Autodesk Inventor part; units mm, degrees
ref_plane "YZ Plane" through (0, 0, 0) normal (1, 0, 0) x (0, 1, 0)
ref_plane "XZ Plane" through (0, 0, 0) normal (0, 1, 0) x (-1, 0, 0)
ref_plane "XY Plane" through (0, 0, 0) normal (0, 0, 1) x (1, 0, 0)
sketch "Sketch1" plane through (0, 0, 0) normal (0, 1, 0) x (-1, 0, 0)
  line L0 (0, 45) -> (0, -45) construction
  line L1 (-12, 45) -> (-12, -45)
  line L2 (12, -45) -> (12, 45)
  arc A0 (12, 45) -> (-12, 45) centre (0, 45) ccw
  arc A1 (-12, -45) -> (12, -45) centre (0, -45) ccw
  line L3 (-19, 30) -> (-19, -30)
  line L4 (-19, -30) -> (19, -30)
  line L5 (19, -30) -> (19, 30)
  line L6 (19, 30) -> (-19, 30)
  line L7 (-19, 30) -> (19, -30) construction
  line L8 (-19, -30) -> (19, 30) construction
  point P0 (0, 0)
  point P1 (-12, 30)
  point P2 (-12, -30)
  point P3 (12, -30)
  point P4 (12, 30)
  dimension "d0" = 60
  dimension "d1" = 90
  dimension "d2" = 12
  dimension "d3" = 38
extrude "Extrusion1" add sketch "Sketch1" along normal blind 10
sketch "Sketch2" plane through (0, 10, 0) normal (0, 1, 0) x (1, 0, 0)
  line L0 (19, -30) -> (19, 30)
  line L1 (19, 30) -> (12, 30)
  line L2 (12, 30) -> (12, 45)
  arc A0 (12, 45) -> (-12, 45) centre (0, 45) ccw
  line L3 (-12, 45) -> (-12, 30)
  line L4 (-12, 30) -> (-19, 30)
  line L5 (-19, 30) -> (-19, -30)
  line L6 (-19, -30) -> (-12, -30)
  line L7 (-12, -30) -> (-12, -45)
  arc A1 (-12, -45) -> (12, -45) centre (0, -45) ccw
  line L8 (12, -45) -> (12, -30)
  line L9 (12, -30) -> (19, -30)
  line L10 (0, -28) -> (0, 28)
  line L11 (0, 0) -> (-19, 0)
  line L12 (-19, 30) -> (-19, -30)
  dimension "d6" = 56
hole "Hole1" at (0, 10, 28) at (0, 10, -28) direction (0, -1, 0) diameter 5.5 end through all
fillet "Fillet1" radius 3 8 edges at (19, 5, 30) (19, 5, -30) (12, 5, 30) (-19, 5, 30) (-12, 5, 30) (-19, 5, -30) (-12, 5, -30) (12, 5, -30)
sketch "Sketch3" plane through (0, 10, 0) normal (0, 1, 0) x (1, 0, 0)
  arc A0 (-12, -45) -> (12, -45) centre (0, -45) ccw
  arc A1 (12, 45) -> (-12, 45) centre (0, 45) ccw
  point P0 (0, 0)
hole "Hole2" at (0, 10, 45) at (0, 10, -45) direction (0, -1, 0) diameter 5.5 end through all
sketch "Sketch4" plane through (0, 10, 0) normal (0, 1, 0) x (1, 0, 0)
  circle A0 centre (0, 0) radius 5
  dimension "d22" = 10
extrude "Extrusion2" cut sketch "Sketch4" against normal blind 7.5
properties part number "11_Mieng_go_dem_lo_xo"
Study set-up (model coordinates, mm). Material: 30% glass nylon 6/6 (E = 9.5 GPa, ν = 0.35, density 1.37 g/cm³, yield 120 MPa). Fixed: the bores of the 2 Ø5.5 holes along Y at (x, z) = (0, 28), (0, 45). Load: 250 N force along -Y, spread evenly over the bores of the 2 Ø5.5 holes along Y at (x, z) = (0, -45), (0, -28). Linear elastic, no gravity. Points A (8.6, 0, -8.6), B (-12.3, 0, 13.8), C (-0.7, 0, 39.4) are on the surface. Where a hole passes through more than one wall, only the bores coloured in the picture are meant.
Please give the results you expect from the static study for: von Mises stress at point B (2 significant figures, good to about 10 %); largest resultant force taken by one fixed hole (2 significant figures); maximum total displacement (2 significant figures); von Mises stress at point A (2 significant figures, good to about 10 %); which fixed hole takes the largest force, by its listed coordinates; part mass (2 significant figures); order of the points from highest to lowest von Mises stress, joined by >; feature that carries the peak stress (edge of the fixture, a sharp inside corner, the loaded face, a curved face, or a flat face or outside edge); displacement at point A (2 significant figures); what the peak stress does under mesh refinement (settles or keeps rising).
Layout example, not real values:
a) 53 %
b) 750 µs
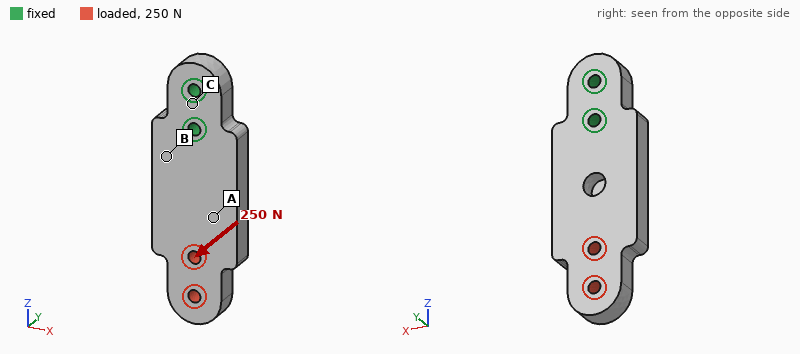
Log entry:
a) 19 MPa
b) 560 N
c) 1.3 mm
d) 11 MPa
e) (0, 28)
f) 45 g
g) B > A > C
h) edge of the fixture
i) 0.38 mm
j) keeps rising
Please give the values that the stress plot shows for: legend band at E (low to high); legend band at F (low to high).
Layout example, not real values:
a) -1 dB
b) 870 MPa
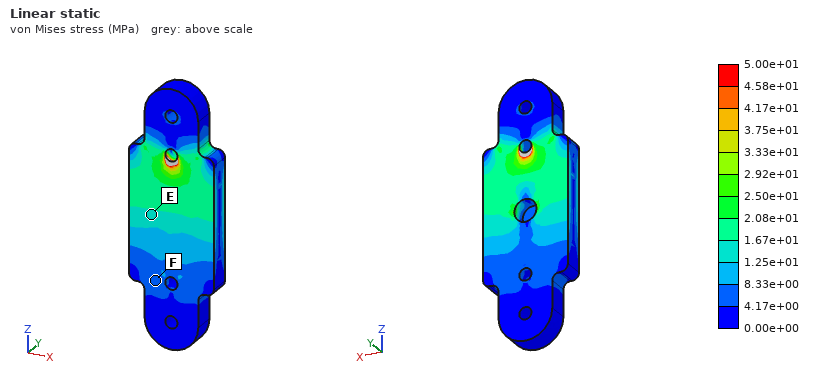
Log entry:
a) 1.25e+01 to 1.67e+01 MPa
b) 4.17e+00 to 8.33e+00 MPa
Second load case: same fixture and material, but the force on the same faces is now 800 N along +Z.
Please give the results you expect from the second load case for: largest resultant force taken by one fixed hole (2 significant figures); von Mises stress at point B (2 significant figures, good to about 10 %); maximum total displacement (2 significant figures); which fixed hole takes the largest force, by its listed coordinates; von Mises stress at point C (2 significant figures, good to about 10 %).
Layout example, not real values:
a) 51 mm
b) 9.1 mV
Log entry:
a) 610 N
b) 2.1 MPa
c) 25 µm
d) (0, 28)
e) 0.63 MPa
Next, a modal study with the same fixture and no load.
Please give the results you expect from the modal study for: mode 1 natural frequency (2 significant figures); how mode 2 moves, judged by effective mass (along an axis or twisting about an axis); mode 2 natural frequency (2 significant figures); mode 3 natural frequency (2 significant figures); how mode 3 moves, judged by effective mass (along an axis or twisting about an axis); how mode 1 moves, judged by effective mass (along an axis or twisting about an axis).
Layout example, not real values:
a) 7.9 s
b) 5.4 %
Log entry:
a) 680 Hz
b) along X
c) 1500 Hz
d) 2700 Hz
e) twisting about Z
f) along Y
